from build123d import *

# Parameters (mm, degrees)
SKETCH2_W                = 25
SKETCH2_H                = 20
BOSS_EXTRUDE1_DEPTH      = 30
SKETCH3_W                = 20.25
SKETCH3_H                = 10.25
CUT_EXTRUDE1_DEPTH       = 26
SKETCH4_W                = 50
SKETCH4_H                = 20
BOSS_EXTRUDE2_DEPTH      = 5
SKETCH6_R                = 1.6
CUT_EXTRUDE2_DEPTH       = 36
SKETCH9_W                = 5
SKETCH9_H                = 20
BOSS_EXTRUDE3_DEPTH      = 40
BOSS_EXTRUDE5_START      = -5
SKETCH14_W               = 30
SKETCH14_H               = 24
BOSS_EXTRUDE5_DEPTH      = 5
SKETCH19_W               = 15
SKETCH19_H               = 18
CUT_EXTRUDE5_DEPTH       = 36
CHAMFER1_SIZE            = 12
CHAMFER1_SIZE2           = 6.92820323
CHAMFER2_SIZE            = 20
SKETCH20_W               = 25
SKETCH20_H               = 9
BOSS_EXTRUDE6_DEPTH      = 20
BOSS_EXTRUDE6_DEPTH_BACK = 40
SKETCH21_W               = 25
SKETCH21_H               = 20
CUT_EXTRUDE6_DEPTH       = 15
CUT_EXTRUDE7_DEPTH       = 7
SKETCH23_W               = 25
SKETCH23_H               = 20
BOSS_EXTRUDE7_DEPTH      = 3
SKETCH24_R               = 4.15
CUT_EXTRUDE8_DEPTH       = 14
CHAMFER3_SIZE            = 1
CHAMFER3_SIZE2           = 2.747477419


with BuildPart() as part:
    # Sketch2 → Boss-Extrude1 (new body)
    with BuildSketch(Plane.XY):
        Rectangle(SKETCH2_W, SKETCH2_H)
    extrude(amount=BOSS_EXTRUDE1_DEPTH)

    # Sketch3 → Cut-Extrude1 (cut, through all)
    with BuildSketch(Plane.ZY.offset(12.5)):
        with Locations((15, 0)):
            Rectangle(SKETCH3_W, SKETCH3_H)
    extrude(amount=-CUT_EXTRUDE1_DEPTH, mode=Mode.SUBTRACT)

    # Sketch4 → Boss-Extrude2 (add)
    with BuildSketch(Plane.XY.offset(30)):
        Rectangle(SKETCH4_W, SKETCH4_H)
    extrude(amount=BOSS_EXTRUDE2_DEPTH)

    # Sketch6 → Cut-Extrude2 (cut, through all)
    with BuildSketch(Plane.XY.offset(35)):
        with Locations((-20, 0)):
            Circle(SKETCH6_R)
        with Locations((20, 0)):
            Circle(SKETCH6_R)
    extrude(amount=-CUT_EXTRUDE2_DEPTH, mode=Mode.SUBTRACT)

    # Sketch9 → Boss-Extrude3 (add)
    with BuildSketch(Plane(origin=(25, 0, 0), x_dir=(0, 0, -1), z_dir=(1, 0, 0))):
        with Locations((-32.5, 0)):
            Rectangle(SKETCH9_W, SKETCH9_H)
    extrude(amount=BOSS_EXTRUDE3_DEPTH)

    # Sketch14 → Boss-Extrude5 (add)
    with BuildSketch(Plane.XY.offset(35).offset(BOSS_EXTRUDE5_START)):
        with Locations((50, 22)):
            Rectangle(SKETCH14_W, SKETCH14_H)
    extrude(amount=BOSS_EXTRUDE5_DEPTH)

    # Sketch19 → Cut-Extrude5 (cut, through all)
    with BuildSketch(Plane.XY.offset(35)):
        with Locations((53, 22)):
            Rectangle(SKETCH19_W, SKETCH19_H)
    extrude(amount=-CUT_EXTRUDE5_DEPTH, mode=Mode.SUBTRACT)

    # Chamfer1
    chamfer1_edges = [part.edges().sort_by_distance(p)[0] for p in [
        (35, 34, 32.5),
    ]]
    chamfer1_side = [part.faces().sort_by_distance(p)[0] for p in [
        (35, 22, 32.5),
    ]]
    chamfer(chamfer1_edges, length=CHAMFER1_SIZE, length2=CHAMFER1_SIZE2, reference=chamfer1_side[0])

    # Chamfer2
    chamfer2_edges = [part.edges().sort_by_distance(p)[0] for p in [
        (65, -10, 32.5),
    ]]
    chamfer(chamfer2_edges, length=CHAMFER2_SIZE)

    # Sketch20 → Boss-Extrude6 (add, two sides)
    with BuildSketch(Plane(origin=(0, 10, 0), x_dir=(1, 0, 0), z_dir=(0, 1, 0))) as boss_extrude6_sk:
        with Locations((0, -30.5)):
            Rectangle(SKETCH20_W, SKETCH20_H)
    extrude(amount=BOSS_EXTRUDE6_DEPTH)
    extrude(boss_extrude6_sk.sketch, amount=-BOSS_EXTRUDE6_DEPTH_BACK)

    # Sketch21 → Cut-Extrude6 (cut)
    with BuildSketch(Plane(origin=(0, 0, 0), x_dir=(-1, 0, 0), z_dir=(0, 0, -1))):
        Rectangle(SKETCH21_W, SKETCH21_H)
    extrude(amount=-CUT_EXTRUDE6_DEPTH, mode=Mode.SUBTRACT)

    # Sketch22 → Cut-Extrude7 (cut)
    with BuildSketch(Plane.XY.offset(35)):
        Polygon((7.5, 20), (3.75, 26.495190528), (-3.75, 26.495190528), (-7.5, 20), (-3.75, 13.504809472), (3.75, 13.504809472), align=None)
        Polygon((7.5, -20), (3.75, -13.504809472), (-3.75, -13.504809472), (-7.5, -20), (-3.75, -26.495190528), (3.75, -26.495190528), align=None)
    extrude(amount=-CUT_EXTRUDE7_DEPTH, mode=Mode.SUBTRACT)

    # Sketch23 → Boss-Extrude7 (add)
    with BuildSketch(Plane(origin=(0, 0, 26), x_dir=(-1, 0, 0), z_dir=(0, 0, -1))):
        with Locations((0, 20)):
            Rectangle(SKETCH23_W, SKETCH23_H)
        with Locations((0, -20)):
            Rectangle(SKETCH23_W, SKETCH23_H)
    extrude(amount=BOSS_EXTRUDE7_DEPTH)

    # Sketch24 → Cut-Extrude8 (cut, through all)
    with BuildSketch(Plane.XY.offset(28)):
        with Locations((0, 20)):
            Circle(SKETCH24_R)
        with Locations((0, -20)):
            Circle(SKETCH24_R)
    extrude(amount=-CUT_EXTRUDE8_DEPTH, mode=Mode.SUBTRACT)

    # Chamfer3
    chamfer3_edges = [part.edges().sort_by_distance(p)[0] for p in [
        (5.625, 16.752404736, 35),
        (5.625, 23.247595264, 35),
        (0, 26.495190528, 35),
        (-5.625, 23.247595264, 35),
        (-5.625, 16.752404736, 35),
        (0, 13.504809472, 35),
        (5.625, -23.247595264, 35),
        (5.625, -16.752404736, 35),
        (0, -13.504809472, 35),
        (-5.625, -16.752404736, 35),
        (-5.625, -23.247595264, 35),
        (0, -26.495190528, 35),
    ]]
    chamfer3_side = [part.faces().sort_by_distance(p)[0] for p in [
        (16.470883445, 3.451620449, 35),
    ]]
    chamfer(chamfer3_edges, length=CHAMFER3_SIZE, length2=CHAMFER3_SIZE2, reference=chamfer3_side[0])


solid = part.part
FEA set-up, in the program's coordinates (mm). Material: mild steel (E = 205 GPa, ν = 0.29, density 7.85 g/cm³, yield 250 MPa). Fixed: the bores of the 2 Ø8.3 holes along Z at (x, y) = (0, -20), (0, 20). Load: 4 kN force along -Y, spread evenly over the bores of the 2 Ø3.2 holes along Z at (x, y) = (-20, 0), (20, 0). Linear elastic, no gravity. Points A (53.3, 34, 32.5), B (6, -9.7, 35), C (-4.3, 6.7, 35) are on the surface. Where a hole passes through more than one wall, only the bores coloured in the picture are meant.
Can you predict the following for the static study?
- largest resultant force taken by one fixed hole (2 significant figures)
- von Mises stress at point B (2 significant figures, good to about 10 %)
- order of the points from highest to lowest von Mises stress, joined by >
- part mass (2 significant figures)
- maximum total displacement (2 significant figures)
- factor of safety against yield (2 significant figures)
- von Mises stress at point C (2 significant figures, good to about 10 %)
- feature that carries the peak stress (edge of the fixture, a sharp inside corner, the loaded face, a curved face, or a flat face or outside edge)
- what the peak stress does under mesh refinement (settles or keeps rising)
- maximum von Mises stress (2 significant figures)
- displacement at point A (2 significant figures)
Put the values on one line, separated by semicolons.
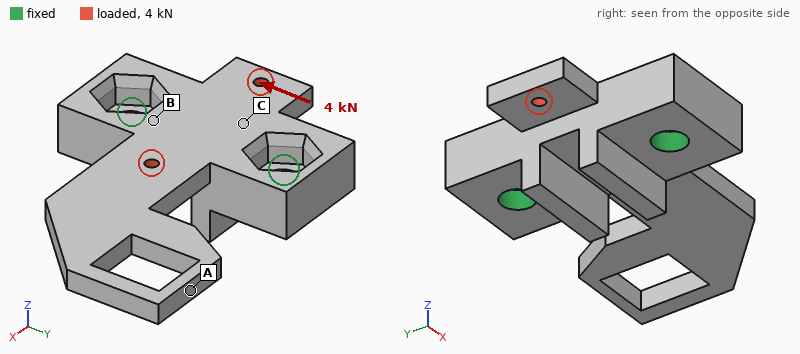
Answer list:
2.1 kN; 22 MPa; B > C > A; 190 g; 16 µm; 2.6; 16 MPa; the loaded face; settles; 97 MPa; 14 µm
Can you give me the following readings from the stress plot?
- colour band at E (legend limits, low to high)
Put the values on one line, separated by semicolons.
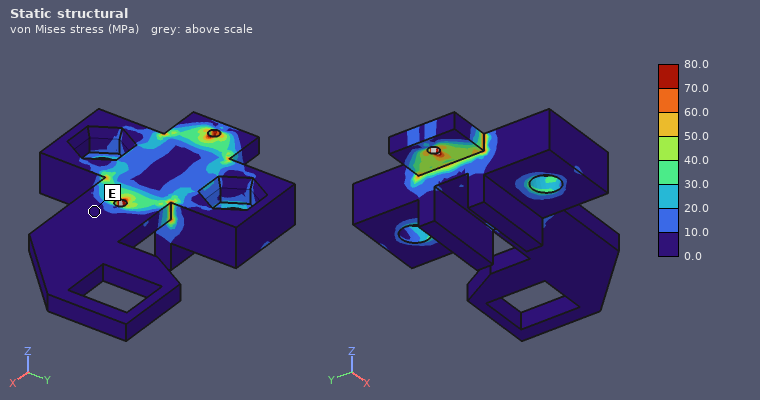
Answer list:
0.0 to 10.0 MPa
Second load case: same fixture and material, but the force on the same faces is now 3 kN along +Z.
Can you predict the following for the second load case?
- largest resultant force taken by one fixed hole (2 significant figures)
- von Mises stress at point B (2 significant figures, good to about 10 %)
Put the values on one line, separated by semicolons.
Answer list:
2.2 kN; 37 MPa
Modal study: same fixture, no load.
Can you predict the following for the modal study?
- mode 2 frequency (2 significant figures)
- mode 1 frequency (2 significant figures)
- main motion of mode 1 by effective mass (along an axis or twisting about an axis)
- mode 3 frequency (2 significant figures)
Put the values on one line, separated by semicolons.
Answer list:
3200 Hz; 1100 Hz; along Z; 3700 Hz
